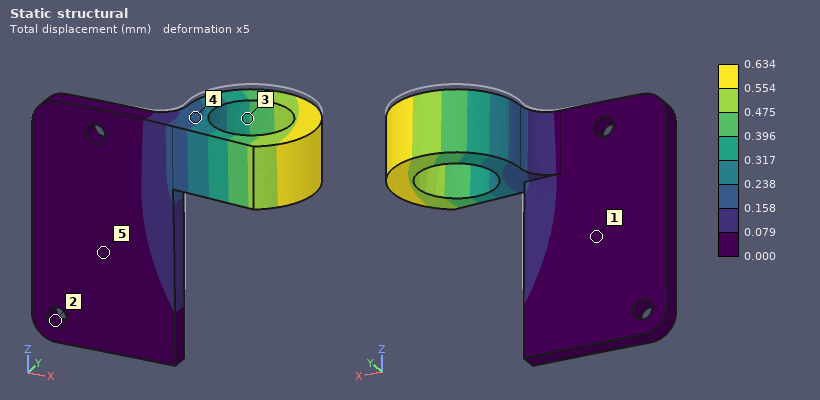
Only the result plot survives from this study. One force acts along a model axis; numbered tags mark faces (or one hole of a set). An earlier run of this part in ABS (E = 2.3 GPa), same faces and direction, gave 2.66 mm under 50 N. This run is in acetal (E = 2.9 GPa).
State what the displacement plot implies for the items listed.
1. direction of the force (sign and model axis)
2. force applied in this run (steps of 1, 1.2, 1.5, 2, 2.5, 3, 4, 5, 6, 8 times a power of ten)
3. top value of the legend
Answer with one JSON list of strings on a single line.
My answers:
["-Y", "15 N", "0.634 mm"]
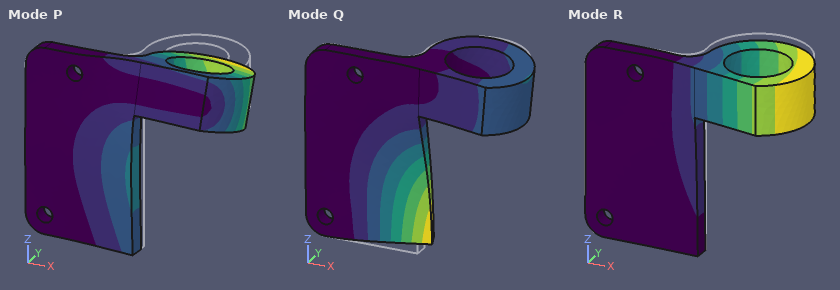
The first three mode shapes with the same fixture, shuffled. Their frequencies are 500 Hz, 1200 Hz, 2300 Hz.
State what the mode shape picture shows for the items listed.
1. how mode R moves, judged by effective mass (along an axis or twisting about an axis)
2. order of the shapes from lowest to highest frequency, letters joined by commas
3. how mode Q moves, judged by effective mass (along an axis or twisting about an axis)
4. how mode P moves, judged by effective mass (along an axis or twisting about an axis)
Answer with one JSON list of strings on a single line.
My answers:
["along Y", "R, P, Q", "along Y", "along Z"]
